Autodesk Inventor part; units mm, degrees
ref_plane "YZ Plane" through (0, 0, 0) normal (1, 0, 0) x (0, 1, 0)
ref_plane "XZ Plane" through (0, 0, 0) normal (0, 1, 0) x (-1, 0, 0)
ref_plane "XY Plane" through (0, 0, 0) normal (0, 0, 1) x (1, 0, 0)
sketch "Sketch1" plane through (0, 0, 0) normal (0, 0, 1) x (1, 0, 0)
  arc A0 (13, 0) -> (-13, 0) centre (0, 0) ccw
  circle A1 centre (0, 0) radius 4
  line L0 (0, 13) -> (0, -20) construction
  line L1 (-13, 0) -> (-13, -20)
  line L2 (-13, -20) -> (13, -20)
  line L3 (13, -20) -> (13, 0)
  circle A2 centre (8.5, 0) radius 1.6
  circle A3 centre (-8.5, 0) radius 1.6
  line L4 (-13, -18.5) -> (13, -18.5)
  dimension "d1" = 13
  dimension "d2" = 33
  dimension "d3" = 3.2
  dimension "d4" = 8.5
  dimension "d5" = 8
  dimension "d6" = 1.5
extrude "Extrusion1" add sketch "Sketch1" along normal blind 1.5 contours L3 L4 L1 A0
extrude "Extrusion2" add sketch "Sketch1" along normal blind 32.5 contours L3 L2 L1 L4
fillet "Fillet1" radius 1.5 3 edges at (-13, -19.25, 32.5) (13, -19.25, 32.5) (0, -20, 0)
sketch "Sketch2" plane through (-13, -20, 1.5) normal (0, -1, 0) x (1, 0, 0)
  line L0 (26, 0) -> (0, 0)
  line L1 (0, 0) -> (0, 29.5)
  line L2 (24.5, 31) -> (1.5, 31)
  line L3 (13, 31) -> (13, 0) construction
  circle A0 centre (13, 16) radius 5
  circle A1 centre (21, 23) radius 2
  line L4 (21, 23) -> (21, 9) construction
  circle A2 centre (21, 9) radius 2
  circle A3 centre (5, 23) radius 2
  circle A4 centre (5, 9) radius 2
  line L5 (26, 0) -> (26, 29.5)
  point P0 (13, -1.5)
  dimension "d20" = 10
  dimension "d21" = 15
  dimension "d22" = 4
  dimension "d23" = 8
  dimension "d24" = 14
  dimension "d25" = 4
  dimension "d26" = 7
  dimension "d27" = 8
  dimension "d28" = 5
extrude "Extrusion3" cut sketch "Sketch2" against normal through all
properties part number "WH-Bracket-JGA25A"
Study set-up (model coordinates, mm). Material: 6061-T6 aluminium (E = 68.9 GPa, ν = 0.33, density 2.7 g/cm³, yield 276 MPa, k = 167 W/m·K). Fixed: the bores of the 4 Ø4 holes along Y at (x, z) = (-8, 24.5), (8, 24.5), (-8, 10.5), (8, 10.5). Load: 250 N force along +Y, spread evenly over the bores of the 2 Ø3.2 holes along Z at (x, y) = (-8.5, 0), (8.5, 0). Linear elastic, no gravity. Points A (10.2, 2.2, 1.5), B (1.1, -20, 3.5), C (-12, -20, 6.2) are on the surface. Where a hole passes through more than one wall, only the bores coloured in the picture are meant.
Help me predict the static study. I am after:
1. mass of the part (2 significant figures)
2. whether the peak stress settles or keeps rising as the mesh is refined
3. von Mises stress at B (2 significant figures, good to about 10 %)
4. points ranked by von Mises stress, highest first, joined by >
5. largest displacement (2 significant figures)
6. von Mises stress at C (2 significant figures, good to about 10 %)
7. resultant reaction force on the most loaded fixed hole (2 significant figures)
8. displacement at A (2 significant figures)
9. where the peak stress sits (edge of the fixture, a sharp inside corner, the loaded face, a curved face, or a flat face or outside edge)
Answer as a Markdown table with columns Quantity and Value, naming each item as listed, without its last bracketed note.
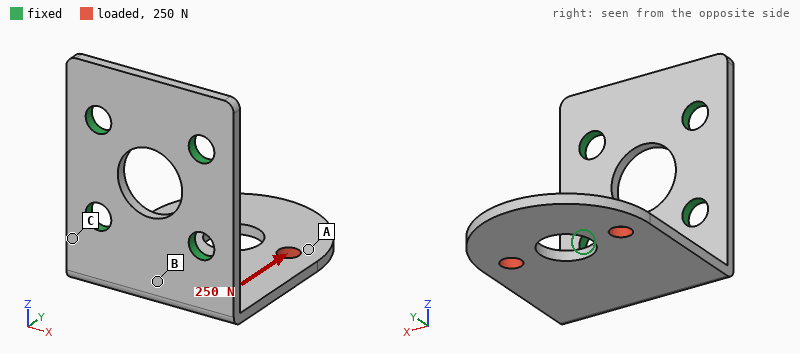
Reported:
| Quantity | Value |
|---|---|
| mass of the part | 5.6 g |
| whether the peak stress settles or keeps rising as the mesh is refined | keeps rising |
| von Mises stress at B | 63 MPa |
| points ranked by von Mises stress, highest first, joined by > | C > B > A |
| largest displacement | 0.58 mm |
| von Mises stress at C | 140 MPa |
| resultant reaction force on the most loaded fixed hole | 130 N |
| displacement at A | 0.39 mm |
| where the peak stress sits | edge of the fixture |
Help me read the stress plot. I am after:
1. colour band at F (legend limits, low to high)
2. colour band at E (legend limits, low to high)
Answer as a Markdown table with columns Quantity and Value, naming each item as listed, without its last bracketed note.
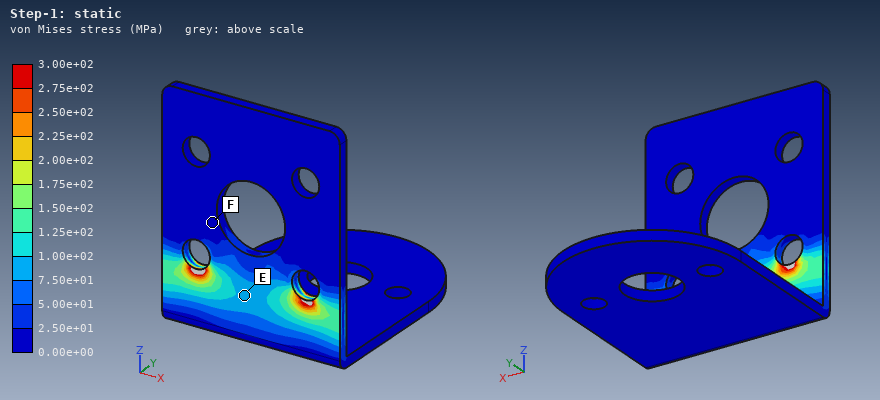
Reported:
| Quantity | Value |
|---|---|
| colour band at F | 0.00e+00 to 2.50e+01 MPa |
| colour band at E | 7.50e+01 to 1.00e+02 MPa |
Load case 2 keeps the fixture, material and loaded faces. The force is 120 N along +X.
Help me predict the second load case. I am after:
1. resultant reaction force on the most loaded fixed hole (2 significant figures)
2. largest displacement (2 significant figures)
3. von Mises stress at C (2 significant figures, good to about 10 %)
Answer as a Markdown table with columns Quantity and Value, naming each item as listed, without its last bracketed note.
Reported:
| Quantity | Value |
|---|---|
| resultant reaction force on the most loaded fixed hole | 150 N |
| largest displacement | 0.23 mm |
| von Mises stress at C | 93 MPa |
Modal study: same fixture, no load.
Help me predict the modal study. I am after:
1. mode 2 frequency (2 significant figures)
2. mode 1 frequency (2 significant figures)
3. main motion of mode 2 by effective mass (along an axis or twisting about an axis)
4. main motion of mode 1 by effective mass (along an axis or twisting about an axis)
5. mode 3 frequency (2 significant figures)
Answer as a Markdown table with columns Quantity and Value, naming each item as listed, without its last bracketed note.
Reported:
| Quantity | Value |
|---|---|
| mode 2 frequency | 2700 Hz |
| mode 1 frequency | 1000 Hz |
| main motion of mode 2 by effective mass | along X |
| main motion of mode 1 by effective mass | along Z |
| mode 3 frequency | 4100 Hz |
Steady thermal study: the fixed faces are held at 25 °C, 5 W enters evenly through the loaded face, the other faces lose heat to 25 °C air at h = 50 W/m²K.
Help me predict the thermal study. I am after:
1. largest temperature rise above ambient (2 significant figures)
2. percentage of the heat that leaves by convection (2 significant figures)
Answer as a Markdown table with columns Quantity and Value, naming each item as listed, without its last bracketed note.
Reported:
| Quantity | Value |
|---|---|
| largest temperature rise above ambient | 21 K |
| percentage of the heat that leaves by convection | 23 % |
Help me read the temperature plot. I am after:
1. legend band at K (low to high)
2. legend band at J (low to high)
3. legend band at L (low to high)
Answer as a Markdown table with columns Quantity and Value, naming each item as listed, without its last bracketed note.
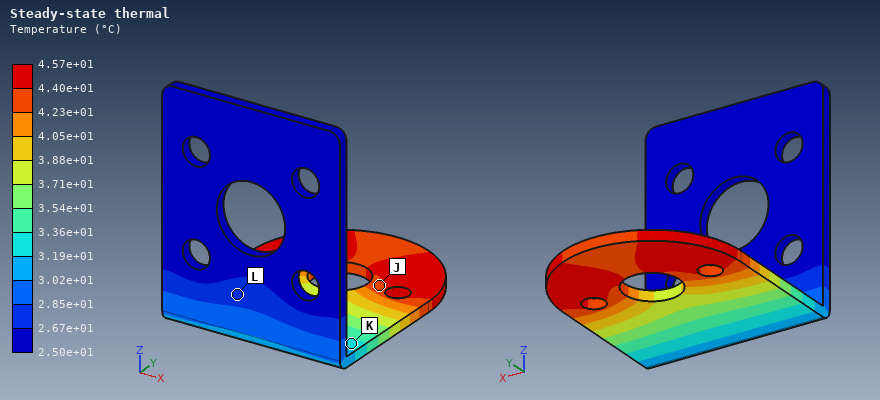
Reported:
| Quantity | Value |
|---|---|
| legend band at K | 3.19e+01 to 3.36e+01 °C |
| legend band at J | 4.23e+01 to 4.40e+01 °C |
| legend band at L | 2.67e+01 to 2.85e+01 °C |
